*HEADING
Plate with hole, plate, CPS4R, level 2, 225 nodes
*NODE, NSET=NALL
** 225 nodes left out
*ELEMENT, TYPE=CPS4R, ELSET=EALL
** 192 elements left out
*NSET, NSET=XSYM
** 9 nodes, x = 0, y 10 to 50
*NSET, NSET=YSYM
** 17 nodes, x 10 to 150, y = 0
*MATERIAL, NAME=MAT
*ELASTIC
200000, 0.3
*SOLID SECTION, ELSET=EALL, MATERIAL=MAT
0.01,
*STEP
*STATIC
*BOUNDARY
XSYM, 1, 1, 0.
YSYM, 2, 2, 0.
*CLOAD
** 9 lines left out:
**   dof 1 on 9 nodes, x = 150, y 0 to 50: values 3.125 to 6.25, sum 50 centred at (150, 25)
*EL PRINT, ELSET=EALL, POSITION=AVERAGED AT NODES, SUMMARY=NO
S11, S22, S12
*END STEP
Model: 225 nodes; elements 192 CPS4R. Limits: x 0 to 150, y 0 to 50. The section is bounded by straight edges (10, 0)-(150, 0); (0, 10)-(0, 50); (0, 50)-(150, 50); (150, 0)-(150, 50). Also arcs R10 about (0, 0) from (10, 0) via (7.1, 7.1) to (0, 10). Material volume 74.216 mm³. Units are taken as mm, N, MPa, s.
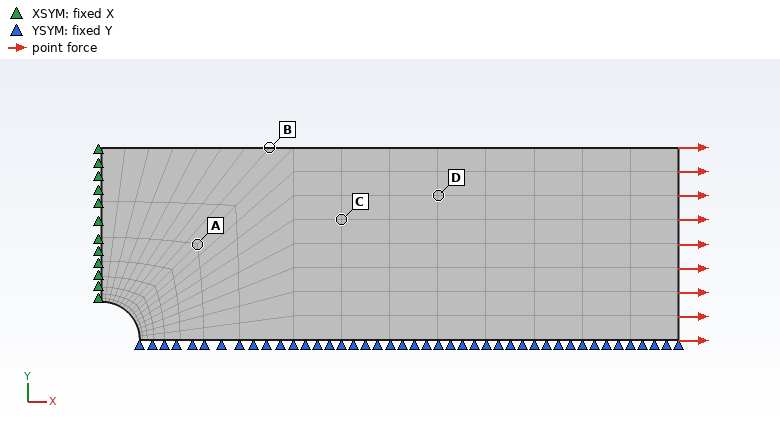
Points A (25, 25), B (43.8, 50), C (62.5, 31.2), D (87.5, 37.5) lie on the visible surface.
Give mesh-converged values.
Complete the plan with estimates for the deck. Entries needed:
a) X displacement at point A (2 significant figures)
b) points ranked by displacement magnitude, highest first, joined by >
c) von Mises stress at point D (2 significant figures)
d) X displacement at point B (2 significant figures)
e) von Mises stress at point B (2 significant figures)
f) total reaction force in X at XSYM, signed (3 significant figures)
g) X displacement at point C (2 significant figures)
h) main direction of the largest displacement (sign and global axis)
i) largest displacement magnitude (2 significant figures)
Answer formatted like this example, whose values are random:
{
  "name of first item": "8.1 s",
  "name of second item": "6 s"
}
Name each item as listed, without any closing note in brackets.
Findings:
{
  "X displacement at point A": "0.014 mm",
  "points ranked by displacement magnitude, highest first, joined by >": "D > C > B > A",
  "von Mises stress at point D": "100 MPa",
  "X displacement at point B": "0.023 mm",
  "von Mises stress at point B": "110 MPa",
  "total reaction force in X at XSYM, signed": "-50.0 N",
  "X displacement at point C": "0.034 mm",
  "main direction of the largest displacement": "+X",
  "largest displacement magnitude": "0.084 mm"
}
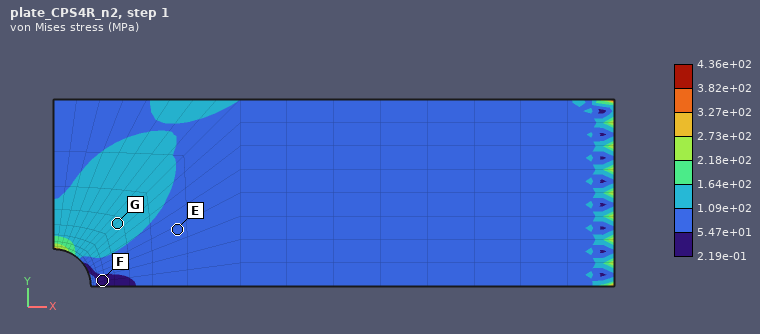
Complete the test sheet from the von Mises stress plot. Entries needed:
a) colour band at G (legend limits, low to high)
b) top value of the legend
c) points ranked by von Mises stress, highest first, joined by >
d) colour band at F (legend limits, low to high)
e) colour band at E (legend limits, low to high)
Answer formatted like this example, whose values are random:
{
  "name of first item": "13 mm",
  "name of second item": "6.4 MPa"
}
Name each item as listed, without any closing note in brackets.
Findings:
{
  "colour band at G": "1.09e+02 to 1.64e+02 MPa",
  "top value of the legend": "4.36e+02 MPa",
  "points ranked by von Mises stress, highest first, joined by >": "G > E > F",
  "colour band at F": "2.19e-01 to 5.47e+01 MPa",
  "colour band at E": "5.47e+01 to 1.09e+02 MPa"
}
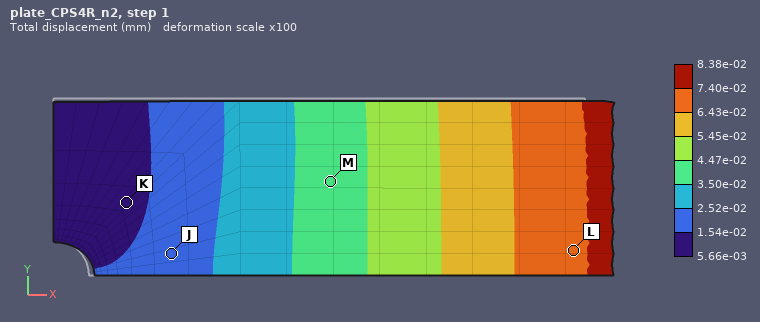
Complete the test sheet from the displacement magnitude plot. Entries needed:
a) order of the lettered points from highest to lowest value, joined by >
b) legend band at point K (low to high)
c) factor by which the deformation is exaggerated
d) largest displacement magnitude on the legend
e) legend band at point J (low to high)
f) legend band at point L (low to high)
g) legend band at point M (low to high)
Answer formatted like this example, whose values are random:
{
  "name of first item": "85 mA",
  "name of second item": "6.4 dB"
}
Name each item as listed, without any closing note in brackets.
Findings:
{
  "order of the lettered points from highest to lowest value, joined by >": "L > M > J > K",
  "legend band at point K": "5.66e-03 to 1.54e-02 mm",
  "factor by which the deformation is exaggerated": "100",
  "largest displacement magnitude on the legend": "8.38e-02 mm",
  "legend band at point J": "1.54e-02 to 2.52e-02 mm",
  "legend band at point L": "6.43e-02 to 7.40e-02 mm",
  "legend band at point M": "3.50e-02 to 4.47e-02 mm"
}
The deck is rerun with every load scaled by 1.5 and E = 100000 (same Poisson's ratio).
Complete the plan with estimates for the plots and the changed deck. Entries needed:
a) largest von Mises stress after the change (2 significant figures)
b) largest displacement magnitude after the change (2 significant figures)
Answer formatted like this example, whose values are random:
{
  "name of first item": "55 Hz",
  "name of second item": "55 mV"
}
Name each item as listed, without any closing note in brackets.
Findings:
{
  "largest von Mises stress after the change": "650 MPa",
  "largest displacement magnitude after the change": "0.25 mm"
}
